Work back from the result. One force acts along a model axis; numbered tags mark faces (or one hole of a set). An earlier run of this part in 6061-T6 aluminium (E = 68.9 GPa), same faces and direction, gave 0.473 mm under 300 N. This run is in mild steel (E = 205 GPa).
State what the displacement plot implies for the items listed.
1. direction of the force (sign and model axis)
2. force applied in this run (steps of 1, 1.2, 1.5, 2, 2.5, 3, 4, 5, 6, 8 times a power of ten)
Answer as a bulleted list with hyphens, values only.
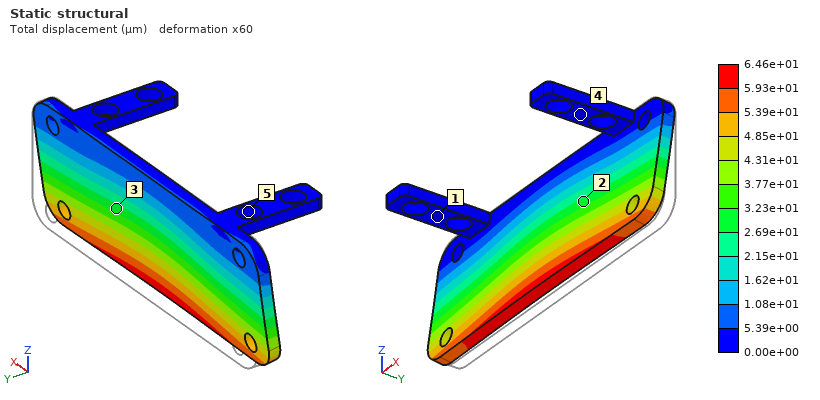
- -Y
- 120 N
